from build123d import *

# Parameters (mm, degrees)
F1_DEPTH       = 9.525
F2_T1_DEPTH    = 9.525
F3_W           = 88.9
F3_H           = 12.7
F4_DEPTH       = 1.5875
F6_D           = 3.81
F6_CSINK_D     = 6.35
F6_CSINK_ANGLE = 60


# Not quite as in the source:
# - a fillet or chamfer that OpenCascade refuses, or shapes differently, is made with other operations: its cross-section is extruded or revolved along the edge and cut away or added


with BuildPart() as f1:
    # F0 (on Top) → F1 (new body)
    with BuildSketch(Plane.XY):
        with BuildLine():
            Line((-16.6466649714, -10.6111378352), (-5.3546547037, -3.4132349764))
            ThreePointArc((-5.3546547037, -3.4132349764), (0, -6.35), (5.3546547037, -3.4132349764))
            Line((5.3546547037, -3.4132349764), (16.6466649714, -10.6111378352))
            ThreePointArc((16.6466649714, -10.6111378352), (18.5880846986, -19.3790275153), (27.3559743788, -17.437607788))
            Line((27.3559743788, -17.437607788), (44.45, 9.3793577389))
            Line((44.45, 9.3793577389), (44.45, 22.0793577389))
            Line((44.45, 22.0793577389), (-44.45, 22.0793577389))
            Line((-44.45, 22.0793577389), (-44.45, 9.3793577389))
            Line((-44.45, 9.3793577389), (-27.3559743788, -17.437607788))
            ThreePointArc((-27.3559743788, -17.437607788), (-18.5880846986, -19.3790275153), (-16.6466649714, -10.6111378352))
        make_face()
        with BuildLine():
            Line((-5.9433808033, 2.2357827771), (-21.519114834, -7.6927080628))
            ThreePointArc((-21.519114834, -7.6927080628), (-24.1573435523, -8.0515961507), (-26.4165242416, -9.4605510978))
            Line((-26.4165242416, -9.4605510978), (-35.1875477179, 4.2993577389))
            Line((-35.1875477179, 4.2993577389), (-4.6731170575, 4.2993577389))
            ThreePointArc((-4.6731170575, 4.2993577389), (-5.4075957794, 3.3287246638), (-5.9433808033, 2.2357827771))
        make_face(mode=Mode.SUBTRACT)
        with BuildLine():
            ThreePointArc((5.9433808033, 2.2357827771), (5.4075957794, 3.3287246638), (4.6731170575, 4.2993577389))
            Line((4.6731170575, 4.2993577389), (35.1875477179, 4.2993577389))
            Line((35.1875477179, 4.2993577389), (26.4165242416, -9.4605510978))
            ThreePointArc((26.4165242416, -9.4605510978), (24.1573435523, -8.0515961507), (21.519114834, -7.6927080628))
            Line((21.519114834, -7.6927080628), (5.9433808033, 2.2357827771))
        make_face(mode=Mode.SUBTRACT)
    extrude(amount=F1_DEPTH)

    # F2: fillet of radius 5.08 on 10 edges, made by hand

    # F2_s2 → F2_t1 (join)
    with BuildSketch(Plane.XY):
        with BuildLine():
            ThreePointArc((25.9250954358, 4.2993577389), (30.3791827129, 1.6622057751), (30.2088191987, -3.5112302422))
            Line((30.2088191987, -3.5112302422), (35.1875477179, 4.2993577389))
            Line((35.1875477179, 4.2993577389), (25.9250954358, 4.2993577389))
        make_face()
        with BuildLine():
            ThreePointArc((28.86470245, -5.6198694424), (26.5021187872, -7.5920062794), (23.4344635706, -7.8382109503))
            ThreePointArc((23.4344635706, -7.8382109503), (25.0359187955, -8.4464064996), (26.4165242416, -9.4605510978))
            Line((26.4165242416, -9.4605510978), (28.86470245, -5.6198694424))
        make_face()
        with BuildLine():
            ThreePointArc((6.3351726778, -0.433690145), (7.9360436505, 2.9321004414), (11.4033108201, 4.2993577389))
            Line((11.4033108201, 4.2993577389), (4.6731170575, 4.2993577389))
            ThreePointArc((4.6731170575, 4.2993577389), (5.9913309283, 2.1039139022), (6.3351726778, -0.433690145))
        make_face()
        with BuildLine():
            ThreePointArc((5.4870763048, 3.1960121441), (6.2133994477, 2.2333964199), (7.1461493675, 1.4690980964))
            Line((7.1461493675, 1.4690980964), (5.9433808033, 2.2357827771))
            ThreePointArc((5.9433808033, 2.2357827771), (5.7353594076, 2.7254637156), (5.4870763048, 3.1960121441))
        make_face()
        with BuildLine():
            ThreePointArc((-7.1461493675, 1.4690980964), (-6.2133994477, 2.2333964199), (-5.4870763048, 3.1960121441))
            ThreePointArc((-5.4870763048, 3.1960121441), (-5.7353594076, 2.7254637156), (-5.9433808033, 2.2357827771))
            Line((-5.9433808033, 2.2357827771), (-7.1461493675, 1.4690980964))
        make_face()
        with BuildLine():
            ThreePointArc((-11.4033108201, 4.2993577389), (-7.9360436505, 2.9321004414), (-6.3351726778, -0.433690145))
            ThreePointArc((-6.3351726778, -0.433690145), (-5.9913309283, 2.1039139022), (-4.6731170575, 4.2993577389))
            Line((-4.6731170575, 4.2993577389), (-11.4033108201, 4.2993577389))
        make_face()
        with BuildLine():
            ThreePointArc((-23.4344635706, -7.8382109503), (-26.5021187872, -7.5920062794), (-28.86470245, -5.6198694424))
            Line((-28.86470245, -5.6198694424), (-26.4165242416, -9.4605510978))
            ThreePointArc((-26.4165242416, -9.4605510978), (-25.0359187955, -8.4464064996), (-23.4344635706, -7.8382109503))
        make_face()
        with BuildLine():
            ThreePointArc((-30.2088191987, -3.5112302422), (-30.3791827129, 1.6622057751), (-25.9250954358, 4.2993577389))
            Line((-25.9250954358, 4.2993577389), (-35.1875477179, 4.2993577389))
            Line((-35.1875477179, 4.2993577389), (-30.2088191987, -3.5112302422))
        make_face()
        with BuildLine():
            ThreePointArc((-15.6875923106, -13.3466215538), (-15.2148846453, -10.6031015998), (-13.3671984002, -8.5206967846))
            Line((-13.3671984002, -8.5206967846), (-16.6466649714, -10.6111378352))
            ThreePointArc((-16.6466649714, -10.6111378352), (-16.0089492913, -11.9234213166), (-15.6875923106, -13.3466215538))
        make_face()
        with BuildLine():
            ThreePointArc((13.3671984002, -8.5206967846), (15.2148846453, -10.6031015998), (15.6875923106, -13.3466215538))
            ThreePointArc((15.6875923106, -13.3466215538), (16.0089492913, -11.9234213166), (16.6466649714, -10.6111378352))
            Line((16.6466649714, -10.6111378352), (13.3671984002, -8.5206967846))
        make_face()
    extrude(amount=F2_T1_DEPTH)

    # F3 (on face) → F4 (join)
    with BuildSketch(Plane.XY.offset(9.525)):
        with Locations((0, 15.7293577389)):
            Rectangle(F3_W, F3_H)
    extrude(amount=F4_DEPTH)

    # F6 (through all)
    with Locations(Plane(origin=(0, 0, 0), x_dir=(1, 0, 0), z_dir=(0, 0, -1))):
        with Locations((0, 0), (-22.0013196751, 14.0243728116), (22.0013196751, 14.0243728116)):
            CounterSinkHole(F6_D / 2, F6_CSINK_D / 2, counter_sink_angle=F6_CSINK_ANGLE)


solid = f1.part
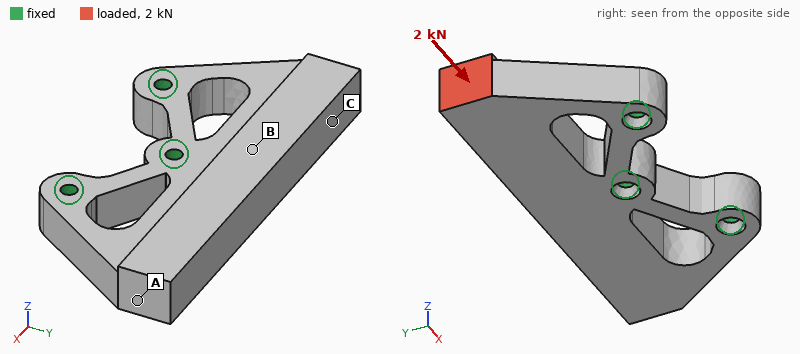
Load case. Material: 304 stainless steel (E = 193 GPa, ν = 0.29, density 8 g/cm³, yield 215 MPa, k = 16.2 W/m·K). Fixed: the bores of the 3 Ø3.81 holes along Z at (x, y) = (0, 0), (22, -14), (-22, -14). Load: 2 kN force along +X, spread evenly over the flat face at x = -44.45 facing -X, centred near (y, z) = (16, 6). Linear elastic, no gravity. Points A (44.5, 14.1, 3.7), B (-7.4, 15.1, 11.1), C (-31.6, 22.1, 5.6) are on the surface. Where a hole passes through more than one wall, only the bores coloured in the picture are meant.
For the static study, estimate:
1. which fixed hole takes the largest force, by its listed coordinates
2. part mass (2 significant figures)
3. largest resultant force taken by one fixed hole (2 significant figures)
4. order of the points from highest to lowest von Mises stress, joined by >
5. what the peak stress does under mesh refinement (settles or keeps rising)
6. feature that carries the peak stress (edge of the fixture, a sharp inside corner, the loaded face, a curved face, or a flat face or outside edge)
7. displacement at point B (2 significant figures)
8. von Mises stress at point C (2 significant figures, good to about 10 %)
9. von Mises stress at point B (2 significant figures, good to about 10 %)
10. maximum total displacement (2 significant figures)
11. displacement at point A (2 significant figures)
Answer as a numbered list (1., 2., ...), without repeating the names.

1. (0, 0)
2. 190 g
3. 1.9 kN
4. C > B > A
5. keeps rising
6. edge of the fixture
7. 3.8 µm
8. 16 MPa
9. 7.5 MPa
10. 8.5 µm
11. 4.2 µm
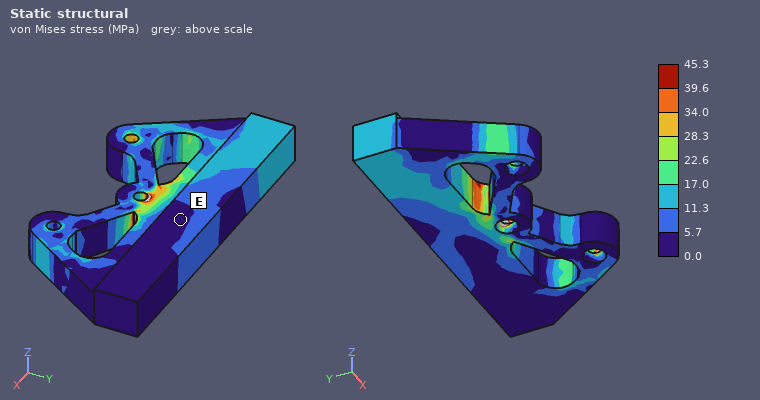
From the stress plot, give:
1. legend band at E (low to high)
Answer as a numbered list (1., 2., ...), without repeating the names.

1. 0.0 to 5.7 MPa
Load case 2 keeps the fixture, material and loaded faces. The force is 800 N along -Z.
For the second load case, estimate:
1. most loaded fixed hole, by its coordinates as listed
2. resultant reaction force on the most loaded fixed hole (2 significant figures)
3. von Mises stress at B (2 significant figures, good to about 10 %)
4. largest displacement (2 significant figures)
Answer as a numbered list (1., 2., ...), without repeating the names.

1. (-22, -14)
2. 590 N
3. 42 MPa
4. 65 µm
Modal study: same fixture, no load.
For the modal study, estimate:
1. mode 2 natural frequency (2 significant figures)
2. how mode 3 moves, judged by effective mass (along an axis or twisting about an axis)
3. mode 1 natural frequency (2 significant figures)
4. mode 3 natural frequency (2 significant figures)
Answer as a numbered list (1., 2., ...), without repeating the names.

1. 4200 Hz
2. along X
3. 4100 Hz
4. 8100 Hz
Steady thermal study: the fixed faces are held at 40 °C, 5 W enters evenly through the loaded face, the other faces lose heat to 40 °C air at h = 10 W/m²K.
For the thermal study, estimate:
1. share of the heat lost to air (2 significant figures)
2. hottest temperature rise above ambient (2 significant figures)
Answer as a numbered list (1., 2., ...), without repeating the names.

1. 20 %
2. 59 K
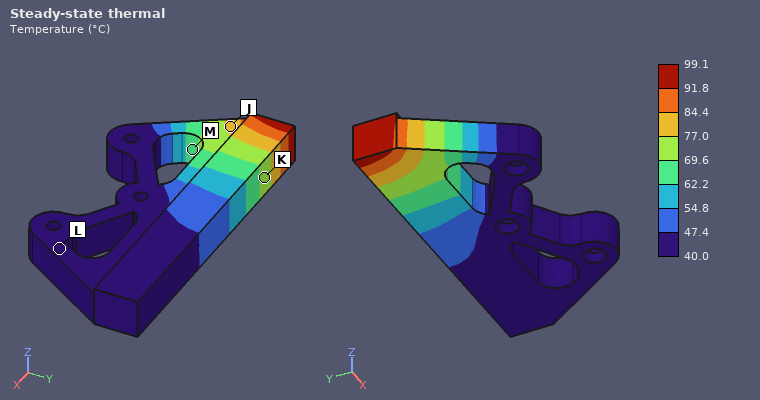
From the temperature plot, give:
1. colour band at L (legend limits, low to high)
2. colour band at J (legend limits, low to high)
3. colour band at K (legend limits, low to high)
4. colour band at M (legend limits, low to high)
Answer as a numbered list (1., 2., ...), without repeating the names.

1. 40.0 to 47.4 °C
2. 77.0 to 84.4 °C
3. 69.6 to 77.0 °C
4. 62.2 to 69.6 °C
